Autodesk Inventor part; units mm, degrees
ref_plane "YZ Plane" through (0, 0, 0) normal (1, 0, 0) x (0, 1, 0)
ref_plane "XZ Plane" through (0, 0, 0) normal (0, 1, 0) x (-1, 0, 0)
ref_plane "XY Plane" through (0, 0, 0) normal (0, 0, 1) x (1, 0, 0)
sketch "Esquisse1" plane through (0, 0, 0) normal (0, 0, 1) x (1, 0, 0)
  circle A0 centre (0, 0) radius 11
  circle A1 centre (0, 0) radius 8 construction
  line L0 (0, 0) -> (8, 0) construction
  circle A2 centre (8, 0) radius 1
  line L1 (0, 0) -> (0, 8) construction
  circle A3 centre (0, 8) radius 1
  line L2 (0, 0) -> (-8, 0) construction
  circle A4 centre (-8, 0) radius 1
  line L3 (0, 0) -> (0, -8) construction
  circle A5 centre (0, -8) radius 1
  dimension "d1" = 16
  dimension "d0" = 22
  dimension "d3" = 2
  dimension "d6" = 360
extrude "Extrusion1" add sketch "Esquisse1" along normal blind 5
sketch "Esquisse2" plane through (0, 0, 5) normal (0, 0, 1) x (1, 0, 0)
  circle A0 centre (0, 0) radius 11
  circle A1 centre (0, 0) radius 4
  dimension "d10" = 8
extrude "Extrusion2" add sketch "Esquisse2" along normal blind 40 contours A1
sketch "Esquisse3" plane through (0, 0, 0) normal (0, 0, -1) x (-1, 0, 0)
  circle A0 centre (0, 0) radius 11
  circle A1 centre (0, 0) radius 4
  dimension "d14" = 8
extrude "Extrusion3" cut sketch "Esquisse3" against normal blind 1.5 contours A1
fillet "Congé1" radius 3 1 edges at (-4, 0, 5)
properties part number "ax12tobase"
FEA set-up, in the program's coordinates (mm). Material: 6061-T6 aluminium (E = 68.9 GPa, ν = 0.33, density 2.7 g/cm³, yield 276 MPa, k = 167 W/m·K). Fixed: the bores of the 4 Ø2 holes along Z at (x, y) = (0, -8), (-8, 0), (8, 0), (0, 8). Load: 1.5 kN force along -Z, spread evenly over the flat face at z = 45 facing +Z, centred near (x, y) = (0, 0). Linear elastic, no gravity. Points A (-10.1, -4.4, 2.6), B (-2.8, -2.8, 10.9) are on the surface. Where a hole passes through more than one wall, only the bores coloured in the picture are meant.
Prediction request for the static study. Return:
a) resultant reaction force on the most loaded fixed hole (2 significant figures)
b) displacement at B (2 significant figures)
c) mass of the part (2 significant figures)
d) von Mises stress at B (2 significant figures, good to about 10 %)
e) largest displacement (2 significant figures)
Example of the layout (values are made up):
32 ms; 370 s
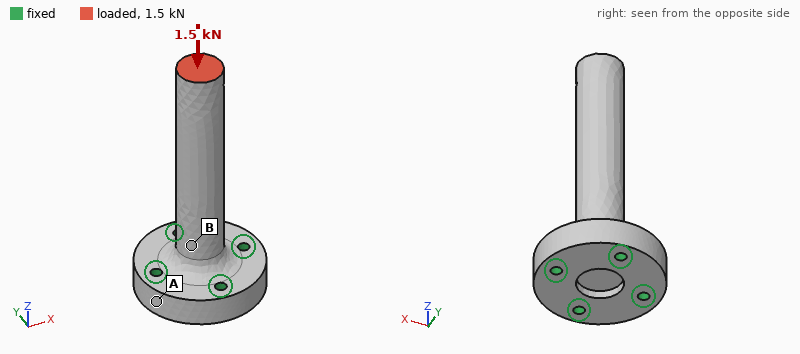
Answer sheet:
410 N; 4.8 µm; 10 g; 29 MPa; 20 µm
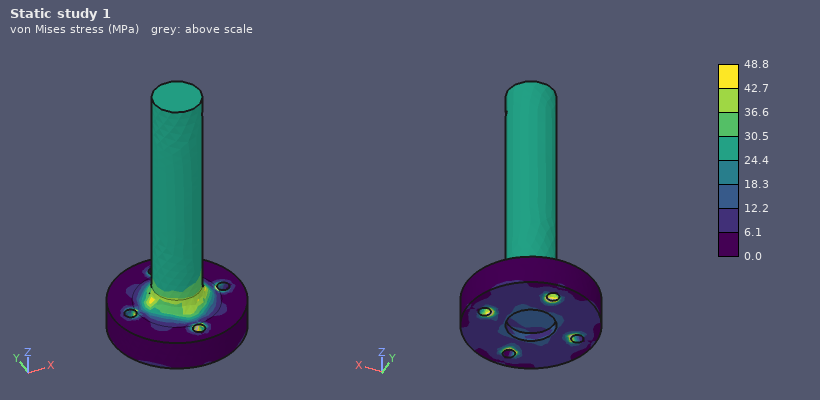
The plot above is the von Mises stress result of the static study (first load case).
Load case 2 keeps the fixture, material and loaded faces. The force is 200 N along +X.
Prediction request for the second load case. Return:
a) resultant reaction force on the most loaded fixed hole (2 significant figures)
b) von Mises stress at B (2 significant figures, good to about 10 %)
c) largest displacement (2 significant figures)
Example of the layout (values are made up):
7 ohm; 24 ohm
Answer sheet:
540 N; 96 MPa; 0.33 mm
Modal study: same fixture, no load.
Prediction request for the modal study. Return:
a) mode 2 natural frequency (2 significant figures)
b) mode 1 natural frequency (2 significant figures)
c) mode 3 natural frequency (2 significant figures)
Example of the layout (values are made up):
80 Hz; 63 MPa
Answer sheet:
3400 Hz; 3400 Hz; 19 kHz
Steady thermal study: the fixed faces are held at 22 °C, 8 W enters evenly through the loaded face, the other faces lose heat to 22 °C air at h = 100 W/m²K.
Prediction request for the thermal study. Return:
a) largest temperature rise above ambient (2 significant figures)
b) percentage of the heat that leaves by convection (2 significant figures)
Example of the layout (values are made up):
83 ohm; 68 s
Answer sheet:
34 K; 22 %
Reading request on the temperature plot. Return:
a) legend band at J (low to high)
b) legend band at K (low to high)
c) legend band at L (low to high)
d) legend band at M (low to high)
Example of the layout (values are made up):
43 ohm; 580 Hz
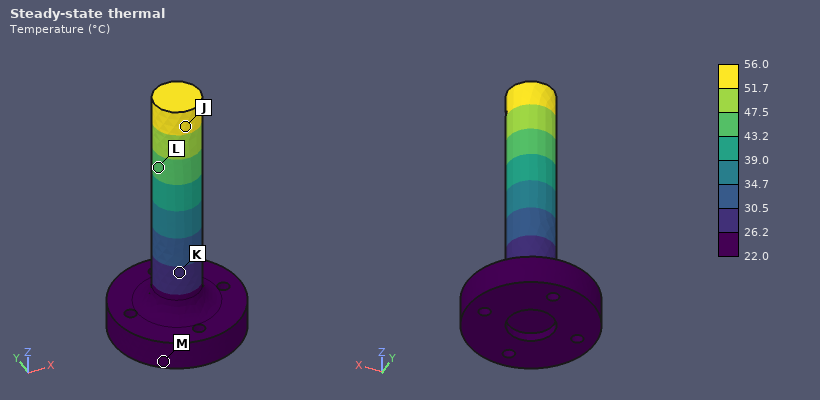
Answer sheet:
51.7 to 56.0 °C; 26.2 to 30.5 °C; 43.2 to 47.5 °C; 22.0 to 26.2 °C
